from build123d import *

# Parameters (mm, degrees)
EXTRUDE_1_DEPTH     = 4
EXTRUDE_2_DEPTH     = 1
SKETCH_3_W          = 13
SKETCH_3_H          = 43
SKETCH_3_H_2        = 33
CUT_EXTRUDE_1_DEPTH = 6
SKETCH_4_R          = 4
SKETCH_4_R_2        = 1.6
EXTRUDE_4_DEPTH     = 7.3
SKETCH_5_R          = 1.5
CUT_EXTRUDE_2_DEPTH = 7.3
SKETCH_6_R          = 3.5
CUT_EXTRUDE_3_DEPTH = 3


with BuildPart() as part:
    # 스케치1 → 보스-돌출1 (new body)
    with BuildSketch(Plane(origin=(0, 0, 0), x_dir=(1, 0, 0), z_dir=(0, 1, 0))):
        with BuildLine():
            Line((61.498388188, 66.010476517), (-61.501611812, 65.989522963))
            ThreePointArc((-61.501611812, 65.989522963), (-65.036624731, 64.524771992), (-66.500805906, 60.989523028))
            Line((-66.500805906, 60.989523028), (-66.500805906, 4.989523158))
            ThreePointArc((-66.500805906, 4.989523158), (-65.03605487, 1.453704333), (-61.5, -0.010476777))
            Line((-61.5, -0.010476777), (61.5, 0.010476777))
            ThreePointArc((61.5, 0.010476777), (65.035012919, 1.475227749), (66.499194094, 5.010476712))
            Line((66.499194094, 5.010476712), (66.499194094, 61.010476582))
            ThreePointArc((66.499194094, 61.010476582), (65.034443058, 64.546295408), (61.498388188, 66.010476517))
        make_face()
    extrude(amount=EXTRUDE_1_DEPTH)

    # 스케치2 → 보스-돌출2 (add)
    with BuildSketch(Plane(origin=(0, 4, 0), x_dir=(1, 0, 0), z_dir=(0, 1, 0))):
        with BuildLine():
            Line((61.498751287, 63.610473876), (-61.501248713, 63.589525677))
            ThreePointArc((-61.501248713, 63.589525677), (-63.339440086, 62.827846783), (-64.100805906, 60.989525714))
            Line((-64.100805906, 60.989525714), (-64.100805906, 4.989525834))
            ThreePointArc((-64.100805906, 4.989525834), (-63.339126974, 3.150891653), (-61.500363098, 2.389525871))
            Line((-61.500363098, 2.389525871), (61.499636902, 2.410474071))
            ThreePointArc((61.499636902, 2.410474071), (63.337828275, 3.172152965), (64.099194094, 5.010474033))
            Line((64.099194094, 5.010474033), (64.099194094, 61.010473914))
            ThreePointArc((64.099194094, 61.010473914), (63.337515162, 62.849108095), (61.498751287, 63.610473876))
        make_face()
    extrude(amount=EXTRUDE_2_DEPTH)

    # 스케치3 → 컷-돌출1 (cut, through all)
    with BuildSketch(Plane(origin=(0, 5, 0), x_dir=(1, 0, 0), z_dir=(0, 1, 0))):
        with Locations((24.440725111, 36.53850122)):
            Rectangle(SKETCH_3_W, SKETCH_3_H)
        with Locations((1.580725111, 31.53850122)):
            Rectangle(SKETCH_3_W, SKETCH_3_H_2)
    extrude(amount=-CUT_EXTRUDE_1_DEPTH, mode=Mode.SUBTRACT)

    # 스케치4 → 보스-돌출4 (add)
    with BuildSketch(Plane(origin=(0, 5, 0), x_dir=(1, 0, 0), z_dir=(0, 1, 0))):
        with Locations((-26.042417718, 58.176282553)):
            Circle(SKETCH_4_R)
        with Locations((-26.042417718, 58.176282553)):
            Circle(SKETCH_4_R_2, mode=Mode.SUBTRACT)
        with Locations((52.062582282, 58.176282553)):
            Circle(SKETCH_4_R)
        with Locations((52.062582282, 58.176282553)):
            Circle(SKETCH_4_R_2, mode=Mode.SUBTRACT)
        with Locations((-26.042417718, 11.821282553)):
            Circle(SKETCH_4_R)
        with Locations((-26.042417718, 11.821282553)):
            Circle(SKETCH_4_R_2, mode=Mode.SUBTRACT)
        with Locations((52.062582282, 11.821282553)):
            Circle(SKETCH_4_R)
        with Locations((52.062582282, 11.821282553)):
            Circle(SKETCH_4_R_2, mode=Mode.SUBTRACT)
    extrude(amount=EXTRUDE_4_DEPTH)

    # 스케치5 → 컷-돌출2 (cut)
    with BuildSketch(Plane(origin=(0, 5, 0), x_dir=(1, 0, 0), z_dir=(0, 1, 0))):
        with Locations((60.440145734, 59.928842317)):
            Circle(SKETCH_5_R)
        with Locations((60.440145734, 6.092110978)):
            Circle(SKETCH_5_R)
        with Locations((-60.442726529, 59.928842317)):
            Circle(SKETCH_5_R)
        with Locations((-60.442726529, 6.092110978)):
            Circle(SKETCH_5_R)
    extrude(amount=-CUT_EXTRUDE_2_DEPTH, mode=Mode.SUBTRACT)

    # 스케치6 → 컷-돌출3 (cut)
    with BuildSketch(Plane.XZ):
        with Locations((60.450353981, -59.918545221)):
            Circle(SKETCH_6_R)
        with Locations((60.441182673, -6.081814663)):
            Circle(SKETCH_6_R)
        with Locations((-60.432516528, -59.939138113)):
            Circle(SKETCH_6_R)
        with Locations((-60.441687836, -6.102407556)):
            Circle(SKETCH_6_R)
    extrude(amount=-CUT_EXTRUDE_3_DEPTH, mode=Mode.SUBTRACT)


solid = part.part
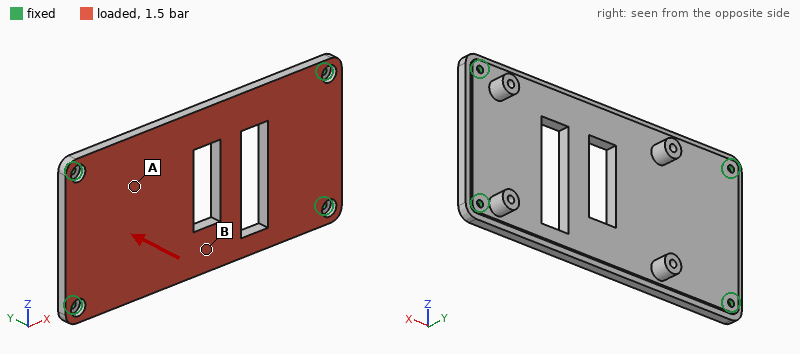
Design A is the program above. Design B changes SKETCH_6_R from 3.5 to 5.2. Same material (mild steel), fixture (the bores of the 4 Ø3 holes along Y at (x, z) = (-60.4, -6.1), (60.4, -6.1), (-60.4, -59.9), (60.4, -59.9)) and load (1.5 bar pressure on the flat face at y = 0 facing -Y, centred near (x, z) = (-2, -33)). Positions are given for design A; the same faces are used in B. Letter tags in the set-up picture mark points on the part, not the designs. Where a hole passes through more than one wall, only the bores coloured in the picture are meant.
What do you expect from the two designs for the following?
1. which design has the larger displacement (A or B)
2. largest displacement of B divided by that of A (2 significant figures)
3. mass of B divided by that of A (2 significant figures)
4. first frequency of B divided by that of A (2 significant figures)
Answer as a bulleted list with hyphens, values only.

- B
- 1.1
- 0.99
- 0.95
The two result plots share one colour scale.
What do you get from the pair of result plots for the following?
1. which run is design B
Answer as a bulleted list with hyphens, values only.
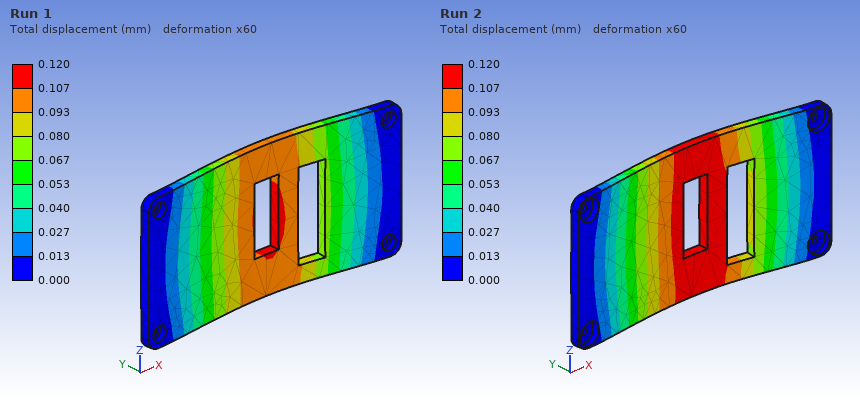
- Run 2
